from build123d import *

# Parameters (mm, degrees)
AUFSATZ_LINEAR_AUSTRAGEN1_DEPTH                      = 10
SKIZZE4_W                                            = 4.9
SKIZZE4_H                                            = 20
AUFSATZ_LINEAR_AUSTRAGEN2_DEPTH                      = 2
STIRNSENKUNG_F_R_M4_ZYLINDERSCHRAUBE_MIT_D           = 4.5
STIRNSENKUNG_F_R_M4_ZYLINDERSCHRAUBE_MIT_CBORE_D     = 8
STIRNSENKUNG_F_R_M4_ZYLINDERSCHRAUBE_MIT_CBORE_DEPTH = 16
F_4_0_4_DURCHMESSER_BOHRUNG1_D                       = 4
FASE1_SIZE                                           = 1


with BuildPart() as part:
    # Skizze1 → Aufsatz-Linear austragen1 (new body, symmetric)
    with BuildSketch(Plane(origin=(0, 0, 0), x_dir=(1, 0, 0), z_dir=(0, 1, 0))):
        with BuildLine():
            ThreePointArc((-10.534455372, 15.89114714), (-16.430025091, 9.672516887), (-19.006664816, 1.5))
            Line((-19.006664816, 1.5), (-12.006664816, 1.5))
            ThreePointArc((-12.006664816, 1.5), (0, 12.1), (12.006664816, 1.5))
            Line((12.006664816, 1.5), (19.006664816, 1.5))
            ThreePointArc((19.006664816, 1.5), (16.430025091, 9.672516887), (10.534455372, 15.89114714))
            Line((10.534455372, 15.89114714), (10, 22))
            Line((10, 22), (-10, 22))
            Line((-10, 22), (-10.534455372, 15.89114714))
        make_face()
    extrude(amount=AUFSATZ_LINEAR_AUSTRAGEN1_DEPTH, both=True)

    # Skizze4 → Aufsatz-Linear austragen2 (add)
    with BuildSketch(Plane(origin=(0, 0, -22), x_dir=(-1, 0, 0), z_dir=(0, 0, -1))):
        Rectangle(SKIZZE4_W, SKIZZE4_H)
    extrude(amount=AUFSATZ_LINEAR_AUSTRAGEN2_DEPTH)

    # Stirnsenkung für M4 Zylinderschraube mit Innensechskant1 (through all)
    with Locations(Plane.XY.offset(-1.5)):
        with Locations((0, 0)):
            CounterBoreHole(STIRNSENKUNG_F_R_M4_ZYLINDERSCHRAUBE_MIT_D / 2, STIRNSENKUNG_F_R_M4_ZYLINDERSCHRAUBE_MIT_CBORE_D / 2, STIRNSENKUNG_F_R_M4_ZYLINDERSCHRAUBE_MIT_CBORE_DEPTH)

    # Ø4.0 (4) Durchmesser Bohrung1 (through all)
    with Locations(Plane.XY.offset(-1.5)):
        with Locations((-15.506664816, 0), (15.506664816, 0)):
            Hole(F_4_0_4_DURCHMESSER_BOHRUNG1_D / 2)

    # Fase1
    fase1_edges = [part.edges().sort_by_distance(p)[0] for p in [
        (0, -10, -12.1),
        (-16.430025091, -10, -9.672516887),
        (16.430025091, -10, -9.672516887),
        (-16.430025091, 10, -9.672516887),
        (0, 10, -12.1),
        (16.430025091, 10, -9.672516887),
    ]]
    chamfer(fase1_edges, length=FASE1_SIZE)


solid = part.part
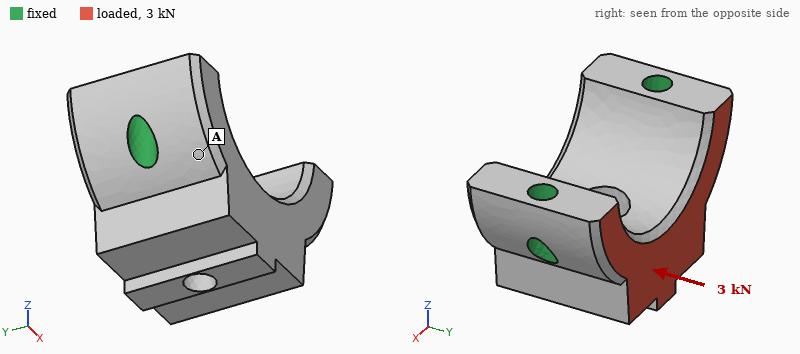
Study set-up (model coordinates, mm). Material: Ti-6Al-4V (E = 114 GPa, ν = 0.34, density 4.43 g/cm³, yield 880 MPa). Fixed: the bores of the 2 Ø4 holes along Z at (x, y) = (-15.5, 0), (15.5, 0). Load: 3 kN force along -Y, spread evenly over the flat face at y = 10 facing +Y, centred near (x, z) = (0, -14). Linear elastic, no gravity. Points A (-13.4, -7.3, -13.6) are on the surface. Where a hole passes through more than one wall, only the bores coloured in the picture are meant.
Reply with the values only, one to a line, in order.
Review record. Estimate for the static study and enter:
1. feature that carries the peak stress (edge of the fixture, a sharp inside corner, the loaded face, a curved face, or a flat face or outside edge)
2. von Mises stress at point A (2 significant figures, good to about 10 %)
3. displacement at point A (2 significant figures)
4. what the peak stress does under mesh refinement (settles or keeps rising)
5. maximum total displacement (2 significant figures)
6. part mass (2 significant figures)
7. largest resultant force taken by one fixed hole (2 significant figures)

edge of the fixture
18 MPa
3.1 µm
keeps rising
12 µm
33 g
1.5 kN
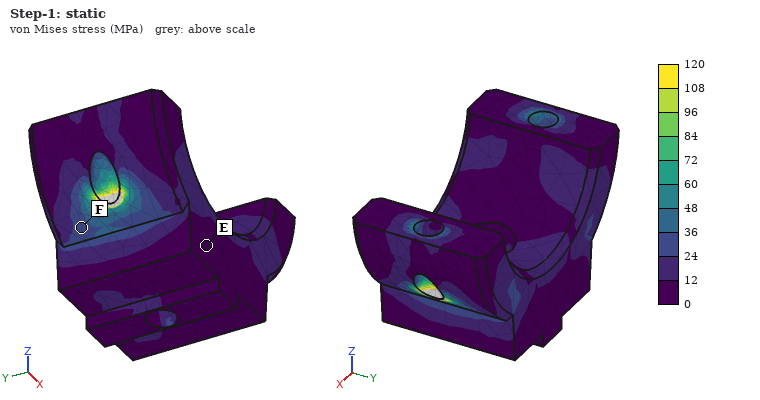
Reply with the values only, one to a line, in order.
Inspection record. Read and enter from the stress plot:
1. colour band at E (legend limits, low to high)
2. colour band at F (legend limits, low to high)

0 to 12 MPa
24 to 36 MPa
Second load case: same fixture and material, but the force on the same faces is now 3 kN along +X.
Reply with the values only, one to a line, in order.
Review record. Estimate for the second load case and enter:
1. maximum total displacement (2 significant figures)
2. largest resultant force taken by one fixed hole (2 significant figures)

6.2 µm
1.8 kN
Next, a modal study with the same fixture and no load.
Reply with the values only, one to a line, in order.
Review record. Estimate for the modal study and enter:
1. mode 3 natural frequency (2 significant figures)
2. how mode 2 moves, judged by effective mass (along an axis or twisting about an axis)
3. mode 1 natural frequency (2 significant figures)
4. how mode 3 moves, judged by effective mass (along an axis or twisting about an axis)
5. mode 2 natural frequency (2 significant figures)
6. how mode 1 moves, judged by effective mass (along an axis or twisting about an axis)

38 kHz
along Z
18 kHz
along X
34 kHz
along Y
